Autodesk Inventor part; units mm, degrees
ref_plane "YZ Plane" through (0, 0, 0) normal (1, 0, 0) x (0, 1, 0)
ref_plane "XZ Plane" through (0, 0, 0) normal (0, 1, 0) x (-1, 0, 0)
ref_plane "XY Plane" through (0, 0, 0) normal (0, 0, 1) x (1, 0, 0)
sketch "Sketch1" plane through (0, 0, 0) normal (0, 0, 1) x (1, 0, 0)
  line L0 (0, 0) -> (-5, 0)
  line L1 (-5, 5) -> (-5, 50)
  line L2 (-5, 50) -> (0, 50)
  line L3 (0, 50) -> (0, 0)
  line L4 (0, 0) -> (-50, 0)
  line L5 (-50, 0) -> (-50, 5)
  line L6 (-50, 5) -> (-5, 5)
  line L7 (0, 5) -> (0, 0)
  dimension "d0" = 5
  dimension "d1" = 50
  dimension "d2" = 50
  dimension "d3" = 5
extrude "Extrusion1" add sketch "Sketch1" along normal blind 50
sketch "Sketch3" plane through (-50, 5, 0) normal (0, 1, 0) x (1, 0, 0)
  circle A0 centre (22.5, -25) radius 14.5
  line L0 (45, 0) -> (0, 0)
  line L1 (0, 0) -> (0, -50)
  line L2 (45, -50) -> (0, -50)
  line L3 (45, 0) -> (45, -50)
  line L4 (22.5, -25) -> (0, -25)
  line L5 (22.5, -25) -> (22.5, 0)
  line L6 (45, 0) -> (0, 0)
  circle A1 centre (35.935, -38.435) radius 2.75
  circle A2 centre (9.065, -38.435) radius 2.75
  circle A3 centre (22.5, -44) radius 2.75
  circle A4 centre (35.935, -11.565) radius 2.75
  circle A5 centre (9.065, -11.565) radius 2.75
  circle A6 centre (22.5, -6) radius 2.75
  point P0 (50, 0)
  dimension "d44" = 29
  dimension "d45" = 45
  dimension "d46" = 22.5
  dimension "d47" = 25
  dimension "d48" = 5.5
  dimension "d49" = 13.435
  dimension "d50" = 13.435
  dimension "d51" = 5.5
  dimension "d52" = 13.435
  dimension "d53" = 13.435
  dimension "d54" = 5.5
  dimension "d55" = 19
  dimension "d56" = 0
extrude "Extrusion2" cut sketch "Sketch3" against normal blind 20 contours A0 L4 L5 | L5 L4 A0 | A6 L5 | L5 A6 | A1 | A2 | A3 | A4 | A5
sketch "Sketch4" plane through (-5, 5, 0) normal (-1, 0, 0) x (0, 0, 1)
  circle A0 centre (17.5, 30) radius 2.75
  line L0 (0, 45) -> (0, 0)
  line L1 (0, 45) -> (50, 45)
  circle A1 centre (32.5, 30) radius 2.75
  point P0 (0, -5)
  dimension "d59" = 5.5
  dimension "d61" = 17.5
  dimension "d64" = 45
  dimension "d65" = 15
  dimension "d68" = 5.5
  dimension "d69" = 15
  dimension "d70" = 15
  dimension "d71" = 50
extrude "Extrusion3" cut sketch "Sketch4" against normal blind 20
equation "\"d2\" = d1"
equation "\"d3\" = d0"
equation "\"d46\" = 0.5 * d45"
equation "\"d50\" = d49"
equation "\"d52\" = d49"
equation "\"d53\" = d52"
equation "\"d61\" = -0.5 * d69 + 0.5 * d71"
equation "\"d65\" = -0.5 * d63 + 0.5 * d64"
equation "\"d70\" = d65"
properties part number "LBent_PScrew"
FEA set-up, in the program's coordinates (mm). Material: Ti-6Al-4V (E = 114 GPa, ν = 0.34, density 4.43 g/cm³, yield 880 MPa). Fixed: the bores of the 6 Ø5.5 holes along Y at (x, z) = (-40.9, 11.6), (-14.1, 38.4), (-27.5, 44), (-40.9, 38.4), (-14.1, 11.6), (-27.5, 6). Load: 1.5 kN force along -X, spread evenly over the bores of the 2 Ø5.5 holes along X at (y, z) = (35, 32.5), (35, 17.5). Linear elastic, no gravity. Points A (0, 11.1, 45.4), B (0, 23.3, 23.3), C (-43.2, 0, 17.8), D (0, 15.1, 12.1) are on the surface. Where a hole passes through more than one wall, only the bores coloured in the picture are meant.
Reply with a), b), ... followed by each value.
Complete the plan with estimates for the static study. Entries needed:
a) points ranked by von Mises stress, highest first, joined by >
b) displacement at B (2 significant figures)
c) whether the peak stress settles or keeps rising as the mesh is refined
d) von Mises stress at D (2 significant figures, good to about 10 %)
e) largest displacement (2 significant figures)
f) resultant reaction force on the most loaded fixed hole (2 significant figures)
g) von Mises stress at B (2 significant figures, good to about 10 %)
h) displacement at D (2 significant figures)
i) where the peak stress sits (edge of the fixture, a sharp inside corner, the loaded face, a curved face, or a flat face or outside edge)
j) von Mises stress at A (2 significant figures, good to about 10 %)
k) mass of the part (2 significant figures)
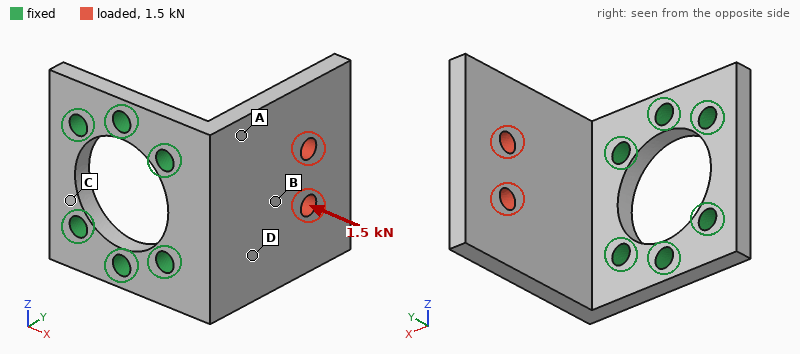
a) A > D > B > C
b) 0.33 mm
c) keeps rising
d) 130 MPa
e) 0.88 mm
f) 960 N
g) 77 MPa
h) 0.19 mm
i) edge of the fixture
j) 170 MPa
k) 86 g
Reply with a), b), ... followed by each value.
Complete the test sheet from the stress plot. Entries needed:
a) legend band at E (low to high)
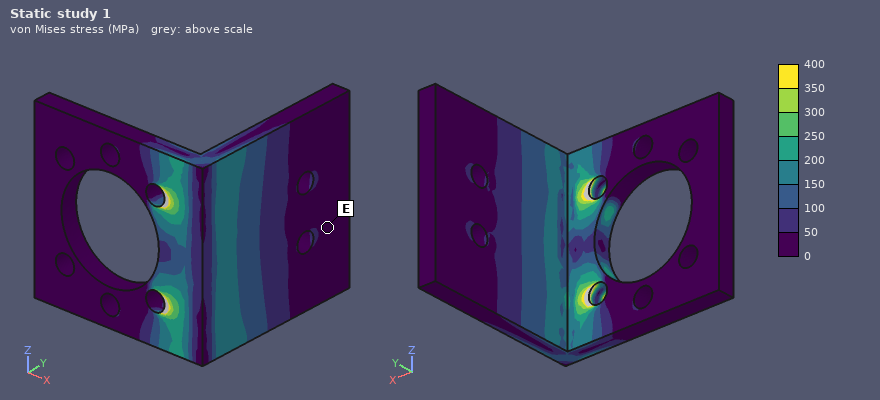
a) 0 to 50 MPa
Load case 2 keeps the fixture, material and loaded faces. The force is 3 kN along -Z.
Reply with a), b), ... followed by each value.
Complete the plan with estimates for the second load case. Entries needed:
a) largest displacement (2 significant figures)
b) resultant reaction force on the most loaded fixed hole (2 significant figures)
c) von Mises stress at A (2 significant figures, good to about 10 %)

a) 0.17 mm
b) 3.7 kN
c) 43 MPa
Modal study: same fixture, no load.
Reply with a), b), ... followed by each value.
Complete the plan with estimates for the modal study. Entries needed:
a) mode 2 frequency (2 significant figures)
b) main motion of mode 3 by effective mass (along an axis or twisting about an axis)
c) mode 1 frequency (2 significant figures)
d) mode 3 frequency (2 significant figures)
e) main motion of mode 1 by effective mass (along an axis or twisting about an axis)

a) 3400 Hz
b) along Z
c) 1400 Hz
d) 4800 Hz
e) along X
